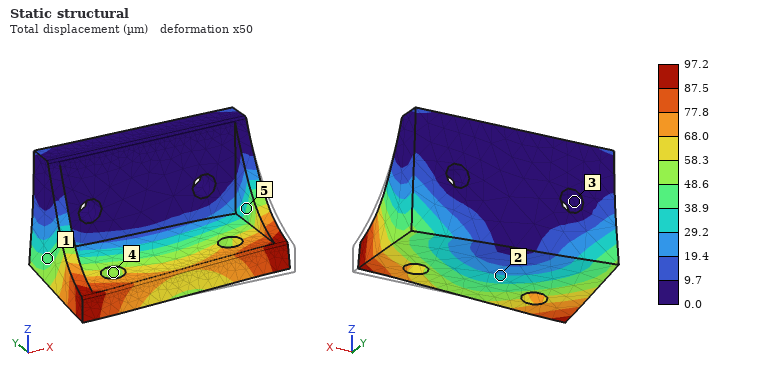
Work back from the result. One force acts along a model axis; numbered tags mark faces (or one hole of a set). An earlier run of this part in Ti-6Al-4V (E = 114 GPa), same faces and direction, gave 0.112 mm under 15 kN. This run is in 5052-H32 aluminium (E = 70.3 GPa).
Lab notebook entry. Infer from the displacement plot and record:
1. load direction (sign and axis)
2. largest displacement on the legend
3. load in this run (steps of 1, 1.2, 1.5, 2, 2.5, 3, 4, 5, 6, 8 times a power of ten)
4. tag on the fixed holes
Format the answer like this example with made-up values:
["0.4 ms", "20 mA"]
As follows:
["-X", "97.2 µm", "8 kN", "3"]
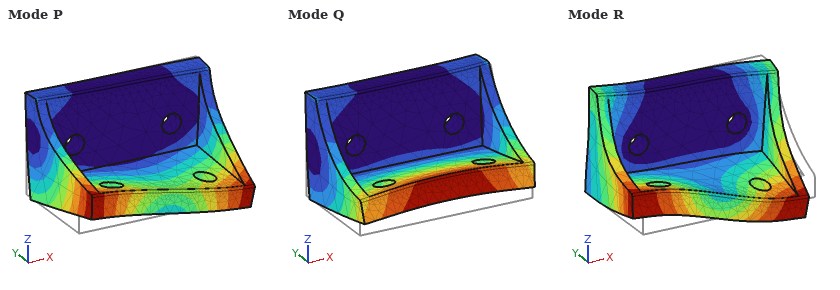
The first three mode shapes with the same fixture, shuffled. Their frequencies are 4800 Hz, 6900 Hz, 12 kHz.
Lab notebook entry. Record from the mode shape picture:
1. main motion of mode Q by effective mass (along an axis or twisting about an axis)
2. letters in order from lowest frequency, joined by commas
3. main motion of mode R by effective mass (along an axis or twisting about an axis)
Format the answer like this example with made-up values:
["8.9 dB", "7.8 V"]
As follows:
["along Z", "Q, P, R", "along X"]
